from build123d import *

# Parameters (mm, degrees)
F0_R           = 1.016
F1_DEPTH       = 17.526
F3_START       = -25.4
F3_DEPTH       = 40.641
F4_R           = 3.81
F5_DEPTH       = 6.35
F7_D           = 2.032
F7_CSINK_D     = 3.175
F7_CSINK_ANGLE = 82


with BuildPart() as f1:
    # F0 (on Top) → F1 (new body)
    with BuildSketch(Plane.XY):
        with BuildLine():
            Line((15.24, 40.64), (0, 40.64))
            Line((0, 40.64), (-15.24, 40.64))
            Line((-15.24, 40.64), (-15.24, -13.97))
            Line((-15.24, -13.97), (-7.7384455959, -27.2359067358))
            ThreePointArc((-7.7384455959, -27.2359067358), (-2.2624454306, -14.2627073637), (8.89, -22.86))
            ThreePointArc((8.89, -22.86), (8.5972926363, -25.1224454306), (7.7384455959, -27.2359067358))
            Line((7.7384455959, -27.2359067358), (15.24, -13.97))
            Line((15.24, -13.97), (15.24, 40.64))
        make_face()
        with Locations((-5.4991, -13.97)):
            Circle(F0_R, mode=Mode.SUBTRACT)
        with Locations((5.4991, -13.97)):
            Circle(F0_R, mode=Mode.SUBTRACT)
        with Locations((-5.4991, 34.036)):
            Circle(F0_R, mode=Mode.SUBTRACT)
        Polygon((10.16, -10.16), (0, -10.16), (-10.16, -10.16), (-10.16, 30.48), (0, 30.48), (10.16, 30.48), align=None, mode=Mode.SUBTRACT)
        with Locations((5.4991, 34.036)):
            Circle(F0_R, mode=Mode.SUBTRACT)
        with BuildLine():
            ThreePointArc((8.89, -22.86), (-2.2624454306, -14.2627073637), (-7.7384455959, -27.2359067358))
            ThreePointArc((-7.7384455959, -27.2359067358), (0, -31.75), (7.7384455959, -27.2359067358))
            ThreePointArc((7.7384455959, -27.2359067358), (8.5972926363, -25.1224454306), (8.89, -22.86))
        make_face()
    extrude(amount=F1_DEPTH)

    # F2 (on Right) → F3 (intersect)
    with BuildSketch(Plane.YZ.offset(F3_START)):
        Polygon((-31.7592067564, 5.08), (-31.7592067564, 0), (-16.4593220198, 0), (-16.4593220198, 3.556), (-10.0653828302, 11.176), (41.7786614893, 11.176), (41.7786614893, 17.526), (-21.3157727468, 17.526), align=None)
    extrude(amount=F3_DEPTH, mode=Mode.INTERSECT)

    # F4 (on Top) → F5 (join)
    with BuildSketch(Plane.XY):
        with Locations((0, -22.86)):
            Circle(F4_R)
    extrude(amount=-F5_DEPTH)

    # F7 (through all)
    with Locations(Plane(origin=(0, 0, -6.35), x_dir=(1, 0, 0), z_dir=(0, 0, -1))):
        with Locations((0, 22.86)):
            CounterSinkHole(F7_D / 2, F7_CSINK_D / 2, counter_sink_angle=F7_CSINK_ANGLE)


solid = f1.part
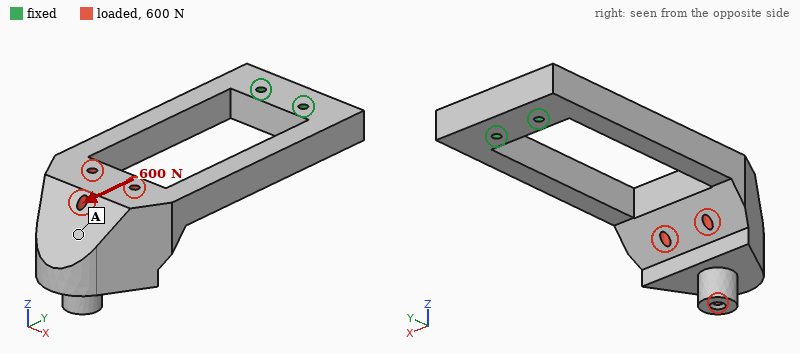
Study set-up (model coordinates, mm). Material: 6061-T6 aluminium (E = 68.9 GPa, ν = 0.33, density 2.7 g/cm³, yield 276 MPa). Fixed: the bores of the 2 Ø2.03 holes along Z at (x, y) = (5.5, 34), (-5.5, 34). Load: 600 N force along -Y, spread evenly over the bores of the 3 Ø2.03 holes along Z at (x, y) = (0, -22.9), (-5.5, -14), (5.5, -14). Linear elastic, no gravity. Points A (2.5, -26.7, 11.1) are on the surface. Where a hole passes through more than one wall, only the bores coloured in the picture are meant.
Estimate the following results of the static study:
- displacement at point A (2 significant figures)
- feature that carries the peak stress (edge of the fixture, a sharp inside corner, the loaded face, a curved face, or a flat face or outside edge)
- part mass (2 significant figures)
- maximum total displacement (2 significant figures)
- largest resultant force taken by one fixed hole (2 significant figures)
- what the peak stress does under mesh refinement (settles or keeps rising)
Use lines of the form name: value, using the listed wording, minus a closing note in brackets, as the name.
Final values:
displacement at point A: 0.46 mm
feature that carries the peak stress: a sharp inside corner
part mass: 29 g
maximum total displacement: 0.54 mm
largest resultant force taken by one fixed hole: 340 N
what the peak stress does under mesh refinement: keeps rising
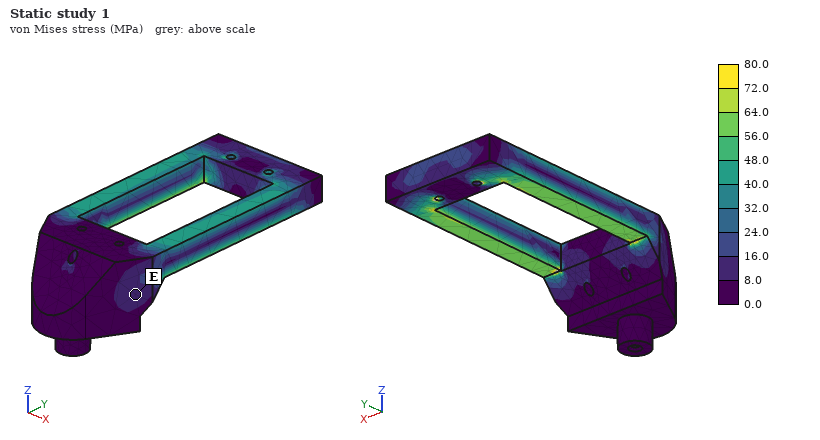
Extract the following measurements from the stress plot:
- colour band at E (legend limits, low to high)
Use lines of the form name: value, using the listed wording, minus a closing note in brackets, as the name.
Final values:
colour band at E: 8.0 to 16.0 MPa
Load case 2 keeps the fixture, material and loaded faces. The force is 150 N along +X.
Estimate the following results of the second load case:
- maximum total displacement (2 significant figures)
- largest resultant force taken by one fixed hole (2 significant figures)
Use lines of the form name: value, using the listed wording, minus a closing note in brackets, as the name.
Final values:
maximum total displacement: 0.22 mm
largest resultant force taken by one fixed hole: 570 N
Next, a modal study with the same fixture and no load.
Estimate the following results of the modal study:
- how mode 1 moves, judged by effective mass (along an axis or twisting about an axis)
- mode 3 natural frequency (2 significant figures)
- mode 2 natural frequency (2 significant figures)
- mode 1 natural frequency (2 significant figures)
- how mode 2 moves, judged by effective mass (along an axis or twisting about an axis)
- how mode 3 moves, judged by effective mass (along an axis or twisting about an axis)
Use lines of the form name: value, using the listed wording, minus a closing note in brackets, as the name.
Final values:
how mode 1 moves, judged by effective mass: along Z
mode 3 natural frequency: 2400 Hz
mode 2 natural frequency: 1000 Hz
mode 1 natural frequency: 580 Hz
how mode 2 moves, judged by effective mass: along X
how mode 3 moves, judged by effective mass: twisting about Y
